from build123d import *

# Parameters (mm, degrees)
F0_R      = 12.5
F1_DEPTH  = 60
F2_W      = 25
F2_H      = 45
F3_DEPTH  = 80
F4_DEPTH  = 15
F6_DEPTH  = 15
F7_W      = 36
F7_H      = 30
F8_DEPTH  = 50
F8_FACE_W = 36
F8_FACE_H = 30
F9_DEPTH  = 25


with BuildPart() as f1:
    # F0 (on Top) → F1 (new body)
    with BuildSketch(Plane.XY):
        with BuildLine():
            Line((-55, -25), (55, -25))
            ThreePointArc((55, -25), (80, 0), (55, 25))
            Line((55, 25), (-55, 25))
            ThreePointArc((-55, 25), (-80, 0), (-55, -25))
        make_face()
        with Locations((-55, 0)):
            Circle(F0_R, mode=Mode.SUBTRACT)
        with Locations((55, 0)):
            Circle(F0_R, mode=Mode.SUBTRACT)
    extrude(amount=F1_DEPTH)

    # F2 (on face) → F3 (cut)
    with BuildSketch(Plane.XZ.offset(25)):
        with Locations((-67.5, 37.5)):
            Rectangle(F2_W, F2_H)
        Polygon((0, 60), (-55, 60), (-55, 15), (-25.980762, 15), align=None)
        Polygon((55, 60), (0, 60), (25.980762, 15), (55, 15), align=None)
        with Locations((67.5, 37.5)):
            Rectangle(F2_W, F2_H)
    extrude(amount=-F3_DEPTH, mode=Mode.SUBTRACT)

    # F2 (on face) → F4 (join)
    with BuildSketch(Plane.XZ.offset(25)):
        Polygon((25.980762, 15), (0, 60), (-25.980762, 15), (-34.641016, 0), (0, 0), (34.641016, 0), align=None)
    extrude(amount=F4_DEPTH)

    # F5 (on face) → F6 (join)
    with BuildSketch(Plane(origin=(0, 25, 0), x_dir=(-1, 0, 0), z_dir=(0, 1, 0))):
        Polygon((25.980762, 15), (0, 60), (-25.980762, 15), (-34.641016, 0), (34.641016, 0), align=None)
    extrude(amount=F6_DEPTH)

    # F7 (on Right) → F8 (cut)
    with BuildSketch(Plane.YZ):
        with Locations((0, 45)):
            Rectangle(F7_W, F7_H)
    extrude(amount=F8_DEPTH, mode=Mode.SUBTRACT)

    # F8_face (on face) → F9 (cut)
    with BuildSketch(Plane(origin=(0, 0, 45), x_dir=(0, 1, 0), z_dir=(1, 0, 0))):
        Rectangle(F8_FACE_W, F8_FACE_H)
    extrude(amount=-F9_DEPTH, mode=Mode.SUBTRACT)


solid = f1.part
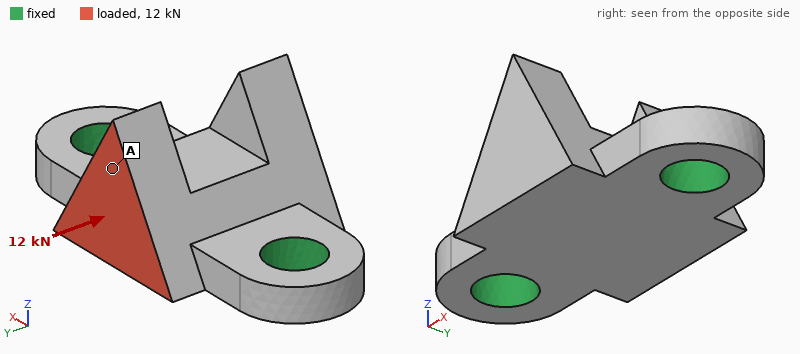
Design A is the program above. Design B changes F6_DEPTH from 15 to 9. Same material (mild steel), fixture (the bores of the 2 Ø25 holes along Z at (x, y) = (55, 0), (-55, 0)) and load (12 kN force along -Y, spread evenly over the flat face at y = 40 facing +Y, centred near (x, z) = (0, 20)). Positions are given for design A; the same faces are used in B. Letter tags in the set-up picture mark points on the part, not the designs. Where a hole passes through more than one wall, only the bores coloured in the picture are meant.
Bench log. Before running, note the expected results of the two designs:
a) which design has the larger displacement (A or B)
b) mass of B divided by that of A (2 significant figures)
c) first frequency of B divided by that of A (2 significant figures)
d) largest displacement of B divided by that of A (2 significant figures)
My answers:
B
0.94
1.1
1.1
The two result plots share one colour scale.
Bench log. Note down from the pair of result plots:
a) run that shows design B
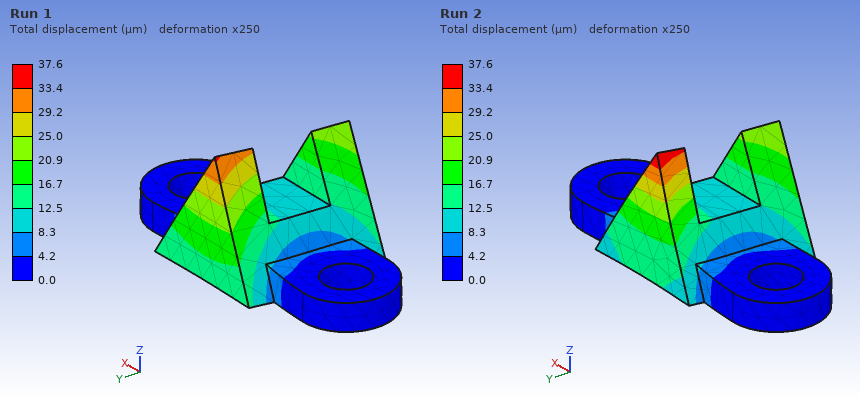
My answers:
Run 2
